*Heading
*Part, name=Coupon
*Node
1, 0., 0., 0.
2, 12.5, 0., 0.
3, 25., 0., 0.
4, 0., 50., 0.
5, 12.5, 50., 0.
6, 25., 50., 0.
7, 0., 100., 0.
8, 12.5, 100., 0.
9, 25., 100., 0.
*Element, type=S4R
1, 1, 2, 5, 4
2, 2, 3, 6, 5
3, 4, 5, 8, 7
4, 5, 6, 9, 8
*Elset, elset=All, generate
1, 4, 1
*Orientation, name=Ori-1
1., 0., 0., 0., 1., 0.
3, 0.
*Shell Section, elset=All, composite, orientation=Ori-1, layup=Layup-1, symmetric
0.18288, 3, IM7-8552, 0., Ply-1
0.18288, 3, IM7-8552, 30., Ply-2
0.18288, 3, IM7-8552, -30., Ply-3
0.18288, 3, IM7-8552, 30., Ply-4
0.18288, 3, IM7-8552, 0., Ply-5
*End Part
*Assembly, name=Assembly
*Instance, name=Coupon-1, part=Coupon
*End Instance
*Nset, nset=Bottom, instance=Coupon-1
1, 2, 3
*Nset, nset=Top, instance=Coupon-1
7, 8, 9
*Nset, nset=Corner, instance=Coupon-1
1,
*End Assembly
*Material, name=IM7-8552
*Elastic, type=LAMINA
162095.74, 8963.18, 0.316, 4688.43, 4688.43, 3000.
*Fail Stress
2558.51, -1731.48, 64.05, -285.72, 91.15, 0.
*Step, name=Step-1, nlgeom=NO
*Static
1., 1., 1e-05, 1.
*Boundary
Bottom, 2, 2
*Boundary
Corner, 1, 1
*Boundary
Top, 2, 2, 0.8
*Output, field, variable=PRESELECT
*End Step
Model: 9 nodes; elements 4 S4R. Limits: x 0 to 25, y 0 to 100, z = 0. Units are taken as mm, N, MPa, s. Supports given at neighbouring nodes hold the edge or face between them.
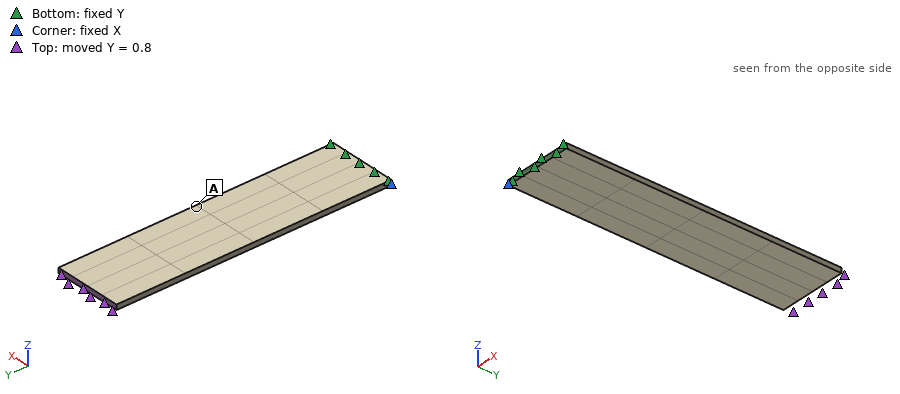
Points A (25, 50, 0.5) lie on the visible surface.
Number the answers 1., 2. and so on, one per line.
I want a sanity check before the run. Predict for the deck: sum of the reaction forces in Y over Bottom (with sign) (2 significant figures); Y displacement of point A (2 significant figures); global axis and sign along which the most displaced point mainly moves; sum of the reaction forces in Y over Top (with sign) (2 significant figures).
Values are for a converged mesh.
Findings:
1. -4500 N
2. 0.40 mm
3. +Y
4. 4500 N
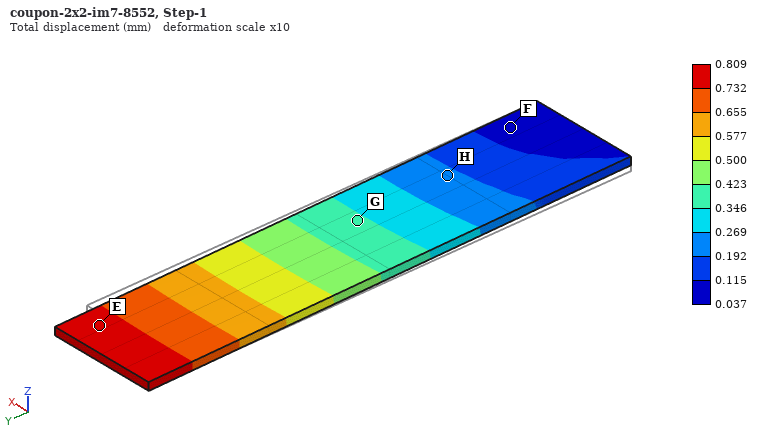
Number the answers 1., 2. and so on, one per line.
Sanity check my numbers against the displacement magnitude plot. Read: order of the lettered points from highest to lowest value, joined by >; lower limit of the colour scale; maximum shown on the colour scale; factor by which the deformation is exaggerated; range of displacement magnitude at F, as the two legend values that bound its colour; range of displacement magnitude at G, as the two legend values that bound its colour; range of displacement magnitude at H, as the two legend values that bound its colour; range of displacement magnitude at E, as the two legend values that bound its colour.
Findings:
1. E > G > H > F
2. 0.037 mm
3. 0.809 mm
4. 10
5. 0.037 to 0.115 mm
6. 0.346 to 0.423 mm
7. 0.192 to 0.269 mm
8. 0.732 to 0.809 mm
